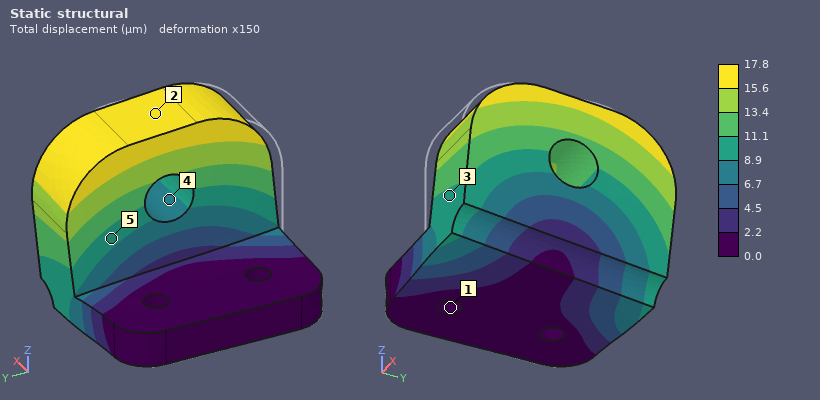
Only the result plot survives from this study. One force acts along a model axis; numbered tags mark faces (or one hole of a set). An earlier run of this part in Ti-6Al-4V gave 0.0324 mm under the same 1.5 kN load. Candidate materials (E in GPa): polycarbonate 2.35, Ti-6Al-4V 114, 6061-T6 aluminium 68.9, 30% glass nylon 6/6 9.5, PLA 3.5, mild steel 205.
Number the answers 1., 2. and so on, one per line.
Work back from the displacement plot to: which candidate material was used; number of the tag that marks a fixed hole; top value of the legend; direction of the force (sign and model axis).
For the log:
1. mild steel
2. 1
3. 17.8 µm
4. +Y
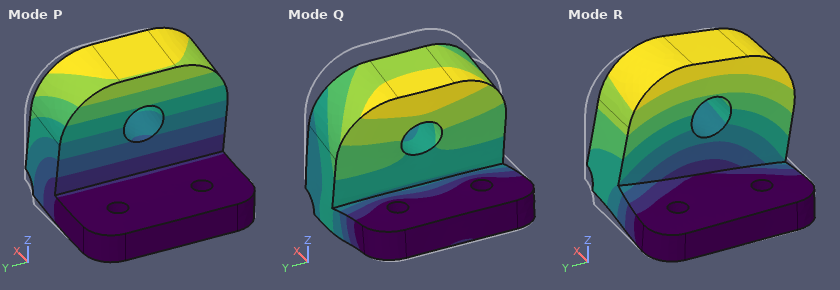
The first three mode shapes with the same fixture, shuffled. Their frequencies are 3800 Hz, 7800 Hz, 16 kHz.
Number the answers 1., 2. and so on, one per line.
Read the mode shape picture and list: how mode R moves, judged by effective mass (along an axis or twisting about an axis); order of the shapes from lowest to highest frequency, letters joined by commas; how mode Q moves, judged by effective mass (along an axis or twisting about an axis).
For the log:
1. along Y
2. P, R, Q
3. along Z
